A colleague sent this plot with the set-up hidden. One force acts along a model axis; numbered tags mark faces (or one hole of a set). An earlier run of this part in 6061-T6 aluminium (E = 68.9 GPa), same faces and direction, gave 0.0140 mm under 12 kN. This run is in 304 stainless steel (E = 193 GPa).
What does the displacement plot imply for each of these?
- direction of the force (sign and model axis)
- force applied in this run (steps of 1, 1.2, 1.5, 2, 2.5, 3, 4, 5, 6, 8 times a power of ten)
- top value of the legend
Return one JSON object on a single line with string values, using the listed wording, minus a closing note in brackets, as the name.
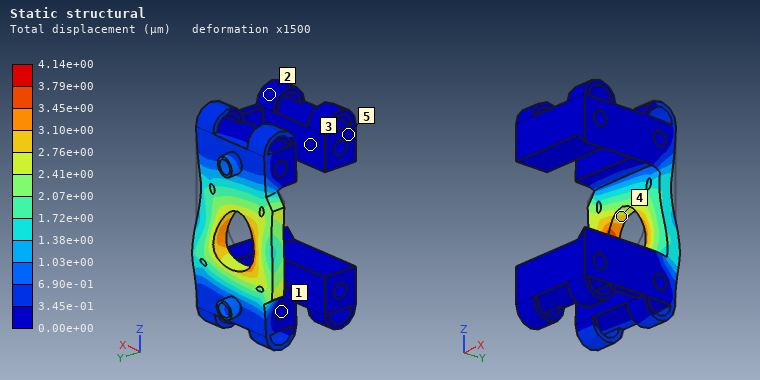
{"direction of the force": "-Z", "force applied in this run": "10 kN", "top value of the legend": "4.14e+00 µm"}
